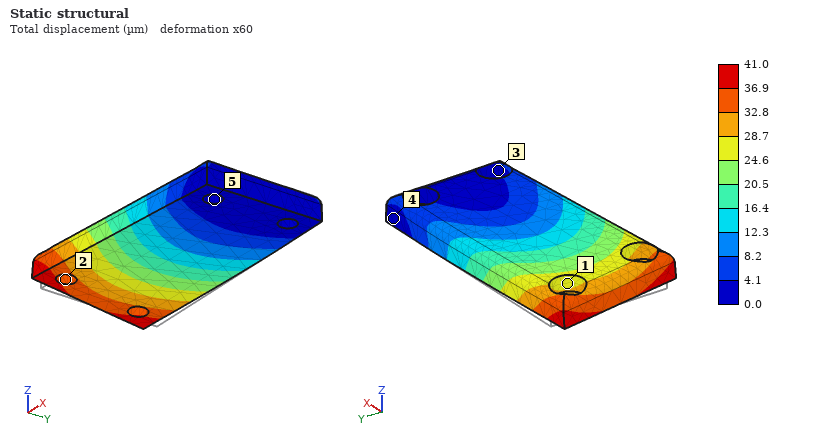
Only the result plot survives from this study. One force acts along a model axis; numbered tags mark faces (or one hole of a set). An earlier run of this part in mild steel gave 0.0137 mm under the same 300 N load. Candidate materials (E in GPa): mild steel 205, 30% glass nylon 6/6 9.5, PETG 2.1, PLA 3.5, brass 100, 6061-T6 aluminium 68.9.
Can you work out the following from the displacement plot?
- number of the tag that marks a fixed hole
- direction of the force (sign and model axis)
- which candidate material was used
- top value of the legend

5
-Y
6061-T6 aluminium
41.0 µm
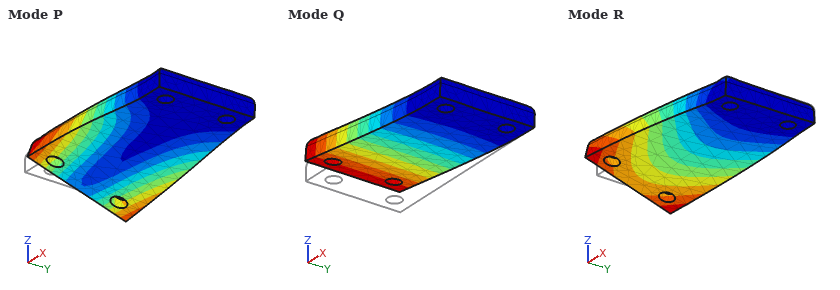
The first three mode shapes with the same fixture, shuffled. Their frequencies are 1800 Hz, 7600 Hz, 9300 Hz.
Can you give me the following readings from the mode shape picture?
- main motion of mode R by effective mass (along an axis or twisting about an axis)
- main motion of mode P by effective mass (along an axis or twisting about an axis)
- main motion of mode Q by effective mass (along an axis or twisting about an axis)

along Y
along Y
along Z
